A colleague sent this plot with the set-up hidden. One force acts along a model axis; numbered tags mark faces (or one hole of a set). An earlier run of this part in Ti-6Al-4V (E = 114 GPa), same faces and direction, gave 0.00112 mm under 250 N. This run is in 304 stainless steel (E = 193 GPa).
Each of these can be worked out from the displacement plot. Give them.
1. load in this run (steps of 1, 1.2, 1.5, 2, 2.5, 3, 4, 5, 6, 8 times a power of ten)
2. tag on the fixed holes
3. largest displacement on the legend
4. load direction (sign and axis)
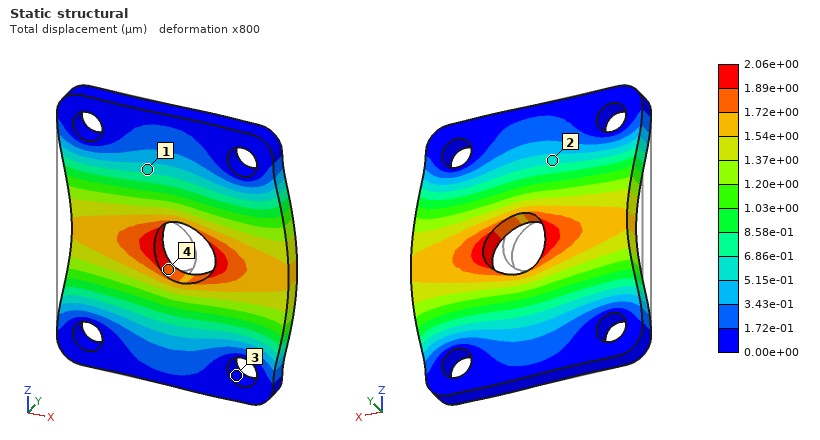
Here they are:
800 N
3
2.06e+00 µm
+X
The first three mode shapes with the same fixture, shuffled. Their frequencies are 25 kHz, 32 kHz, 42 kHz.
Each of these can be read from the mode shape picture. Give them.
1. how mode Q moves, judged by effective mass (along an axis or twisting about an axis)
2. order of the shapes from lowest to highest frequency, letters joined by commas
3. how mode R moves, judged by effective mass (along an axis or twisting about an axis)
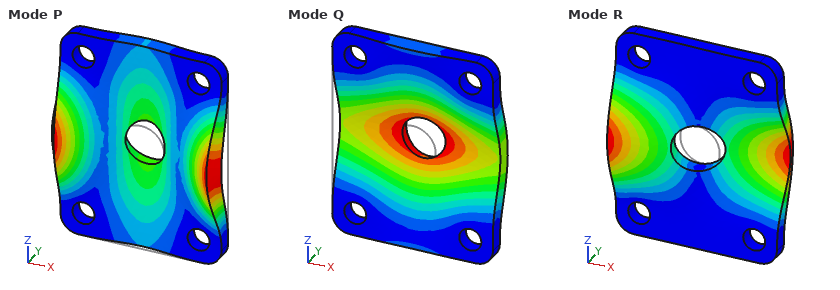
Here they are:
along Y
Q, R, P
twisting about Z
